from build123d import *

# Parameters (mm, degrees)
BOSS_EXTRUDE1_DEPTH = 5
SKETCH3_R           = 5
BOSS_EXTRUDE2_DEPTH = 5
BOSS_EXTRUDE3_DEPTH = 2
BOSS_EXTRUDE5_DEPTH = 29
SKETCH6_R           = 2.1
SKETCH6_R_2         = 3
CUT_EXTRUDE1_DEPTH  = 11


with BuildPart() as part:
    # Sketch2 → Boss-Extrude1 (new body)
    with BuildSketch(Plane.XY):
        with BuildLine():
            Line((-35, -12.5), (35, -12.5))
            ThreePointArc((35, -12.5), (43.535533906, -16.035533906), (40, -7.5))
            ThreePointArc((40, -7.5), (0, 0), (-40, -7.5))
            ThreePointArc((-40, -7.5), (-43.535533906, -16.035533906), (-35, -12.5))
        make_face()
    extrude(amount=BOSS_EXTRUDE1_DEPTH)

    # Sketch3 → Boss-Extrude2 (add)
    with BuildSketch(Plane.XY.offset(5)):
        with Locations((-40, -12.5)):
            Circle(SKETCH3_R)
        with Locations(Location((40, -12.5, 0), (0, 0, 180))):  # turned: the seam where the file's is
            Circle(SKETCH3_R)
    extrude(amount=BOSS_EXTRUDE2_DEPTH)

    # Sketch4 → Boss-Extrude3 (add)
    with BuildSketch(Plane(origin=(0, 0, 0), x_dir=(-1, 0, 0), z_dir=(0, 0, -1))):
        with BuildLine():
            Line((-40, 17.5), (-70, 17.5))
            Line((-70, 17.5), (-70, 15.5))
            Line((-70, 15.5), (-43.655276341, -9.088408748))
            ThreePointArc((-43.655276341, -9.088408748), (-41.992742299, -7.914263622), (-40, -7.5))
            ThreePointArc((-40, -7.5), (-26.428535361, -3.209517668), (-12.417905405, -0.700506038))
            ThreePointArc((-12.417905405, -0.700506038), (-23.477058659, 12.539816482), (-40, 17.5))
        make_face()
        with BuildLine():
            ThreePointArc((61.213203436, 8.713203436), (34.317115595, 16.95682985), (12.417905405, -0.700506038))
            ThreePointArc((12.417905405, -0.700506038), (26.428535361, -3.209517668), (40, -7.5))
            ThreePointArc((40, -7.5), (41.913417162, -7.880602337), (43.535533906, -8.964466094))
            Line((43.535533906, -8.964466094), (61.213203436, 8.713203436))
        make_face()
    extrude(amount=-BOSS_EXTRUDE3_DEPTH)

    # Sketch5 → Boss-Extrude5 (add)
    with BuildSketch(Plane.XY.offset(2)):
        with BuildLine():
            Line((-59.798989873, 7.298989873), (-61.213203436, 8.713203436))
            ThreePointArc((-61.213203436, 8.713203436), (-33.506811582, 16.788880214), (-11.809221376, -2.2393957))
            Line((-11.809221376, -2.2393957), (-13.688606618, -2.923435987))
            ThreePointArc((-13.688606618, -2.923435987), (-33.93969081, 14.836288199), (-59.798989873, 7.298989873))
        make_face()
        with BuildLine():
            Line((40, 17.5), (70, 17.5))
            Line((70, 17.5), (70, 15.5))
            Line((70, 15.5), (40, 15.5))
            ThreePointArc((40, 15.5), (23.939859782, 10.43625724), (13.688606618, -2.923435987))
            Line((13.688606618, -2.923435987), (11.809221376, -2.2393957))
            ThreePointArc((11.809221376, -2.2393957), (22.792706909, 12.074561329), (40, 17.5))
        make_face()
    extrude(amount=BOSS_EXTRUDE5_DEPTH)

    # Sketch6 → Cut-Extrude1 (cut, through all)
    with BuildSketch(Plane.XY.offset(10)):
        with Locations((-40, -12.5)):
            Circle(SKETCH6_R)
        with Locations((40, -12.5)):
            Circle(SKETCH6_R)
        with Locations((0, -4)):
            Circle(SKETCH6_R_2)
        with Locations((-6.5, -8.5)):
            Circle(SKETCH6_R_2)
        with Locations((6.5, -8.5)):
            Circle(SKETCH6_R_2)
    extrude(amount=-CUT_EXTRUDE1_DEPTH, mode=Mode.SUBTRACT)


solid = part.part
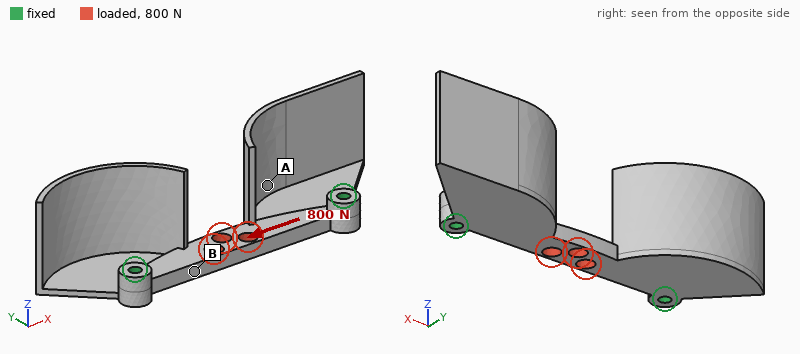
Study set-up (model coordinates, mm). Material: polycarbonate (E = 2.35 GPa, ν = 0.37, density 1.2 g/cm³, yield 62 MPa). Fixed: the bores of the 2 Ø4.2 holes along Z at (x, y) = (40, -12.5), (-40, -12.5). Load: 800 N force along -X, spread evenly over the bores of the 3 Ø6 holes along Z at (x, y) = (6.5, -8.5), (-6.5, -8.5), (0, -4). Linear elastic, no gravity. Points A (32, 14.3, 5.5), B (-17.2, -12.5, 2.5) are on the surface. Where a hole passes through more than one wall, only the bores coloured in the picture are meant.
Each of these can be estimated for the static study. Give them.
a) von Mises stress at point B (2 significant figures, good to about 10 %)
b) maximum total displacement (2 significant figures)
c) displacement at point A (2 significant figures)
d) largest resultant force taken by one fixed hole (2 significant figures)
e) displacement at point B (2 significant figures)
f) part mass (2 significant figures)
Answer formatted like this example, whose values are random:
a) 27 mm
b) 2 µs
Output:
a) 12 MPa
b) 0.23 mm
c) 0.16 mm
d) 400 N
e) 0.13 mm
f) 18 g
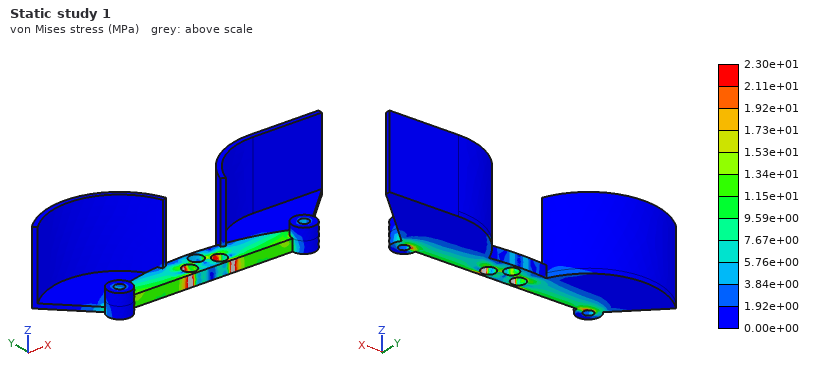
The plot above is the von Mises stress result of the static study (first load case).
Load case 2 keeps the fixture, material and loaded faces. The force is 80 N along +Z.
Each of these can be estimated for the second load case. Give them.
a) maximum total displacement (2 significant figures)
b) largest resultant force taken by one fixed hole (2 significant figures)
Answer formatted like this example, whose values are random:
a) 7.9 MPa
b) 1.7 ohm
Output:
a) 1.4 mm
b) 41 N
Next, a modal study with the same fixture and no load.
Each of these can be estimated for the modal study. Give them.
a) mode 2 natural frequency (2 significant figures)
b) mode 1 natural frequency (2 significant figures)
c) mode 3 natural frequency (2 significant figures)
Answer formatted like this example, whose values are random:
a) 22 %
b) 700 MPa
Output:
a) 310 Hz
b) 250 Hz
c) 340 Hz
